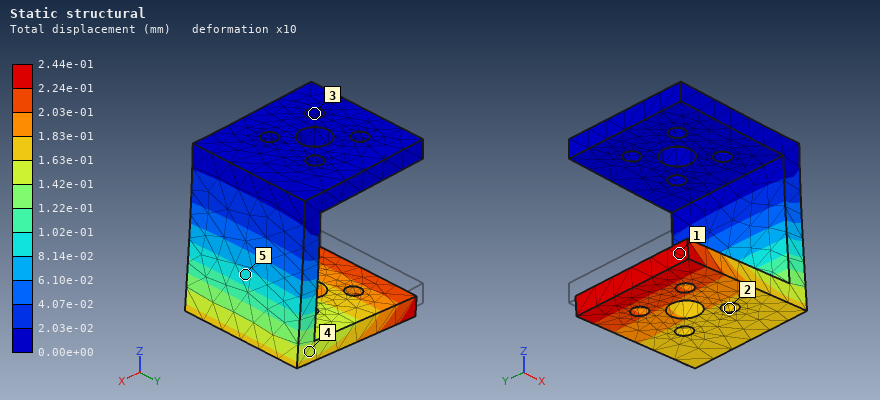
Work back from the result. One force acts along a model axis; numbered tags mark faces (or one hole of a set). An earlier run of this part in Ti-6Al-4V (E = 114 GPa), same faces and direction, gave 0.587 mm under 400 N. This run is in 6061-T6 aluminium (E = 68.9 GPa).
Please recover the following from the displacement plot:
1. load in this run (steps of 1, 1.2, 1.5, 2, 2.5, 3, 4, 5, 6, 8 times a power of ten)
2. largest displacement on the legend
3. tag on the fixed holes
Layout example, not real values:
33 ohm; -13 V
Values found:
100 N; 2.44e-01 mm; 3
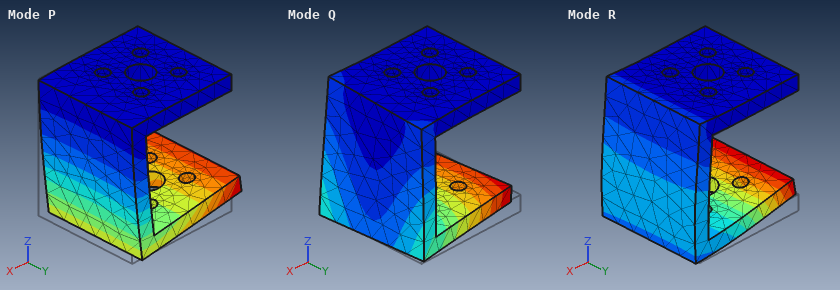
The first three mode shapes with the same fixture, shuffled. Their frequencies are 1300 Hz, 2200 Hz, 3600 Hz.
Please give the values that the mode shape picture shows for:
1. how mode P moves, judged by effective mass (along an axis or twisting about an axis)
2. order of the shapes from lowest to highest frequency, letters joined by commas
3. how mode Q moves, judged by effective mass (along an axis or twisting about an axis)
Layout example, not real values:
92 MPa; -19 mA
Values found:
along X; P, Q, R; along Y
